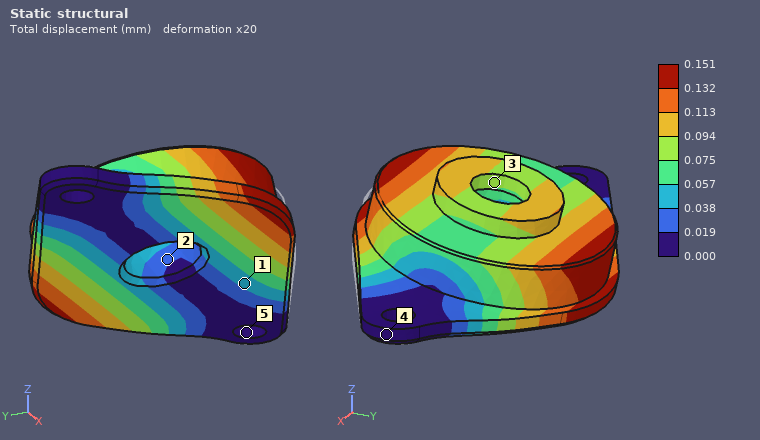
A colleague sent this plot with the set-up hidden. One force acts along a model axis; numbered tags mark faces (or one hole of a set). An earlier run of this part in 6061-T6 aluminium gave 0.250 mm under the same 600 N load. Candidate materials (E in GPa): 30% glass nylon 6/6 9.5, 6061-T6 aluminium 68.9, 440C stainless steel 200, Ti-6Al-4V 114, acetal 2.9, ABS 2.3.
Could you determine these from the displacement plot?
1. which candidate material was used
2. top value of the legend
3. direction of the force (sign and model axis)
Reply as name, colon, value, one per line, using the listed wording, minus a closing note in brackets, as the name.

which candidate material was used: Ti-6Al-4V
top value of the legend: 0.151 mm
direction of the force: +Y
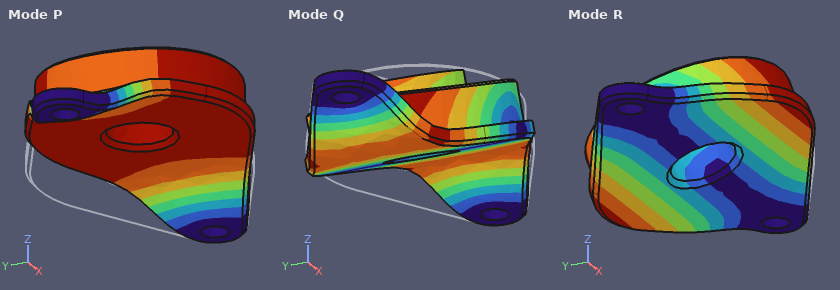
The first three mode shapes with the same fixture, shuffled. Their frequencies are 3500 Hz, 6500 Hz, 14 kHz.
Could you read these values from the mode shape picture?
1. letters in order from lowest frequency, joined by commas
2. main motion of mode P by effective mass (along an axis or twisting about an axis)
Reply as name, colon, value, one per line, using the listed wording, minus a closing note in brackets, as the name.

letters in order from lowest frequency, joined by commas: R, P, Q
main motion of mode P by effective mass: along Z
